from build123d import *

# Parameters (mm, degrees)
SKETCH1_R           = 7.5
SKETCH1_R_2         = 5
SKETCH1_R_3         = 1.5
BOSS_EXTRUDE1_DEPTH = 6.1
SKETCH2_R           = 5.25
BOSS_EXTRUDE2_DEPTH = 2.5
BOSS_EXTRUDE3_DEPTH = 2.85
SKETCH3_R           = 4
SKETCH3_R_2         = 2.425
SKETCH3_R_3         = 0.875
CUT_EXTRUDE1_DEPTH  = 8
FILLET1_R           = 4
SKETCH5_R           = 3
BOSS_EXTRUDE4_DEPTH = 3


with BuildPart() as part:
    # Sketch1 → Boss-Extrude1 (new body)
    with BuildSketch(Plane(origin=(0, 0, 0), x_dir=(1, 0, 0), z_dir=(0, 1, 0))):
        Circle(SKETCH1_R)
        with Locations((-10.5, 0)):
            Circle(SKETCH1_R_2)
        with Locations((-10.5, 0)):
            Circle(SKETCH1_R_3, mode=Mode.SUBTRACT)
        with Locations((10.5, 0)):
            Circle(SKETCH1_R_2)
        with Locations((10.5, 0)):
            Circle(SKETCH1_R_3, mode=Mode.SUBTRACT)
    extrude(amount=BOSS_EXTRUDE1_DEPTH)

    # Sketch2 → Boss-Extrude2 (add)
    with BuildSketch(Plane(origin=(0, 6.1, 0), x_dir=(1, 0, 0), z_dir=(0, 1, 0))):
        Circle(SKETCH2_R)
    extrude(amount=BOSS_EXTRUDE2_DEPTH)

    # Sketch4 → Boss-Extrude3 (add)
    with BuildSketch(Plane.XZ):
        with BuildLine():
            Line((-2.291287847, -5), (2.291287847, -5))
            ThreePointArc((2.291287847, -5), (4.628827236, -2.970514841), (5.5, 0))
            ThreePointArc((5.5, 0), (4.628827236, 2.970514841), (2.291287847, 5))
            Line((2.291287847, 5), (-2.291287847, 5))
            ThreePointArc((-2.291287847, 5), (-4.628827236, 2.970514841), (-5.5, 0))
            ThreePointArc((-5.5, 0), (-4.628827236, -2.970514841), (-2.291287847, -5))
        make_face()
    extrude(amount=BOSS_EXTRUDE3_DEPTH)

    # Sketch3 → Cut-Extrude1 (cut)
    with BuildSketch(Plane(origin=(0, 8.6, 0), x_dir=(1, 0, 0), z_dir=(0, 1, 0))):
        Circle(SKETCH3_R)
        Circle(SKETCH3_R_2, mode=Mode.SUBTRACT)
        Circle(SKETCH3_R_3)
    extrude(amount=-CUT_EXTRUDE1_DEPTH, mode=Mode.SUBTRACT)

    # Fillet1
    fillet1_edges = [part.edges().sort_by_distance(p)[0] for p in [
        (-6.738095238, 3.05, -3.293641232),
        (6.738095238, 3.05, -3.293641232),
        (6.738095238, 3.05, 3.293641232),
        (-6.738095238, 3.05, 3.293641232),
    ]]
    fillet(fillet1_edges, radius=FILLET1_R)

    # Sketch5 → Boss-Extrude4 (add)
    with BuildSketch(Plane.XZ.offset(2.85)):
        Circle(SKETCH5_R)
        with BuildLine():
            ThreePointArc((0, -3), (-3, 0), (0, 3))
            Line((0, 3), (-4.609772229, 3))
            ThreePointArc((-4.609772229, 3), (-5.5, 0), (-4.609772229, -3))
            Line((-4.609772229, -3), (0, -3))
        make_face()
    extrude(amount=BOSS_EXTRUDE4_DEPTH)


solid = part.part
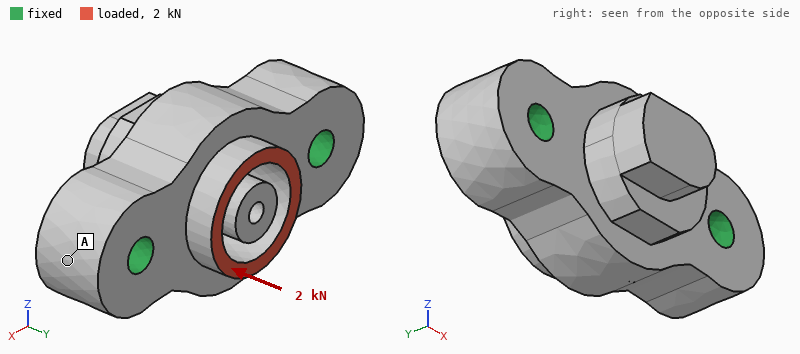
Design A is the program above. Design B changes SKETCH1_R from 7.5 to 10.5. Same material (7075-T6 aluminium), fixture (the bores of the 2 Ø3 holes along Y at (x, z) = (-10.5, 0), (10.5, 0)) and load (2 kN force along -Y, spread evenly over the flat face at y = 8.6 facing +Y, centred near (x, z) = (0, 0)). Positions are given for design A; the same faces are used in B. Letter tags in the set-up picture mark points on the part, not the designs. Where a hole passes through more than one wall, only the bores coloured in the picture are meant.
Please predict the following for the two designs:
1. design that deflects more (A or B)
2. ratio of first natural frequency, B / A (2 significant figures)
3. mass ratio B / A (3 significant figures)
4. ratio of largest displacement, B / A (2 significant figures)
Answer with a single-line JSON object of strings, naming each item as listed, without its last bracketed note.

{"design that deflects more": "A", "ratio of first natural frequency, B / A": "0.89", "mass ratio B / A": "1.31", "ratio of largest displacement, B / A": "0.83"}
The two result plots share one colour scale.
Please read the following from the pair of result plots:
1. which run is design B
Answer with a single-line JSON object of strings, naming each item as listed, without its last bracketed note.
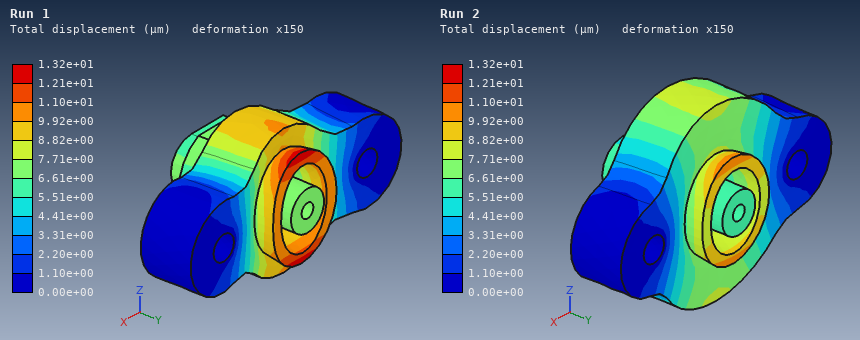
{"which run is design B": "Run 2"}
